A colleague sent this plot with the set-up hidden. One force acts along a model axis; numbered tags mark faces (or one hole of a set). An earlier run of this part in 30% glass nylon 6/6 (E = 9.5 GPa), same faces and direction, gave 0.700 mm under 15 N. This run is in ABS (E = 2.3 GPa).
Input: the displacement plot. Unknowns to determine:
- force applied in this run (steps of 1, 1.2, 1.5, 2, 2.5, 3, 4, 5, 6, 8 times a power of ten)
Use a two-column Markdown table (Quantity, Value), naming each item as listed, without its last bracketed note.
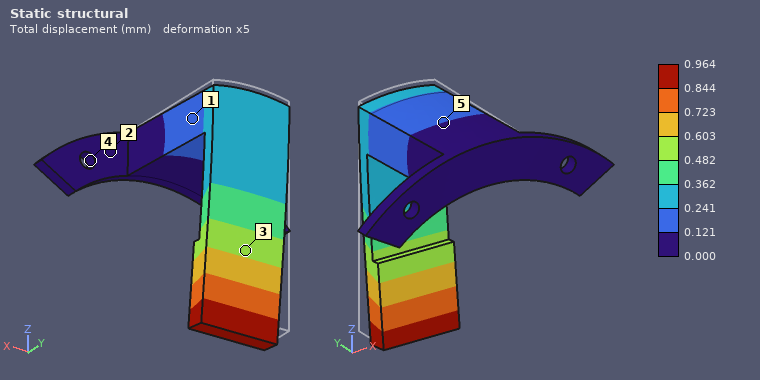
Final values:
| Quantity | Value |
|---|---|
| force applied in this run | 5 N |
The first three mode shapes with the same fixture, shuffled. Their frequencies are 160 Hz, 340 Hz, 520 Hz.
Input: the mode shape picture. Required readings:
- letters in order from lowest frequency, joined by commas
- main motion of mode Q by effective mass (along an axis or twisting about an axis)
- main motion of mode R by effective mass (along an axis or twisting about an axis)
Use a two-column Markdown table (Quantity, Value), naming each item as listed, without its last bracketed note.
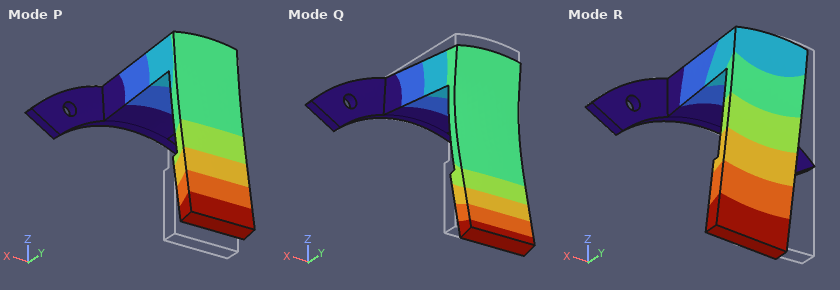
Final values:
| Quantity | Value |
|---|---|
| letters in order from lowest frequency, joined by commas | P, Q, R |
| main motion of mode Q by effective mass | along Z |
| main motion of mode R by effective mass | along X |
